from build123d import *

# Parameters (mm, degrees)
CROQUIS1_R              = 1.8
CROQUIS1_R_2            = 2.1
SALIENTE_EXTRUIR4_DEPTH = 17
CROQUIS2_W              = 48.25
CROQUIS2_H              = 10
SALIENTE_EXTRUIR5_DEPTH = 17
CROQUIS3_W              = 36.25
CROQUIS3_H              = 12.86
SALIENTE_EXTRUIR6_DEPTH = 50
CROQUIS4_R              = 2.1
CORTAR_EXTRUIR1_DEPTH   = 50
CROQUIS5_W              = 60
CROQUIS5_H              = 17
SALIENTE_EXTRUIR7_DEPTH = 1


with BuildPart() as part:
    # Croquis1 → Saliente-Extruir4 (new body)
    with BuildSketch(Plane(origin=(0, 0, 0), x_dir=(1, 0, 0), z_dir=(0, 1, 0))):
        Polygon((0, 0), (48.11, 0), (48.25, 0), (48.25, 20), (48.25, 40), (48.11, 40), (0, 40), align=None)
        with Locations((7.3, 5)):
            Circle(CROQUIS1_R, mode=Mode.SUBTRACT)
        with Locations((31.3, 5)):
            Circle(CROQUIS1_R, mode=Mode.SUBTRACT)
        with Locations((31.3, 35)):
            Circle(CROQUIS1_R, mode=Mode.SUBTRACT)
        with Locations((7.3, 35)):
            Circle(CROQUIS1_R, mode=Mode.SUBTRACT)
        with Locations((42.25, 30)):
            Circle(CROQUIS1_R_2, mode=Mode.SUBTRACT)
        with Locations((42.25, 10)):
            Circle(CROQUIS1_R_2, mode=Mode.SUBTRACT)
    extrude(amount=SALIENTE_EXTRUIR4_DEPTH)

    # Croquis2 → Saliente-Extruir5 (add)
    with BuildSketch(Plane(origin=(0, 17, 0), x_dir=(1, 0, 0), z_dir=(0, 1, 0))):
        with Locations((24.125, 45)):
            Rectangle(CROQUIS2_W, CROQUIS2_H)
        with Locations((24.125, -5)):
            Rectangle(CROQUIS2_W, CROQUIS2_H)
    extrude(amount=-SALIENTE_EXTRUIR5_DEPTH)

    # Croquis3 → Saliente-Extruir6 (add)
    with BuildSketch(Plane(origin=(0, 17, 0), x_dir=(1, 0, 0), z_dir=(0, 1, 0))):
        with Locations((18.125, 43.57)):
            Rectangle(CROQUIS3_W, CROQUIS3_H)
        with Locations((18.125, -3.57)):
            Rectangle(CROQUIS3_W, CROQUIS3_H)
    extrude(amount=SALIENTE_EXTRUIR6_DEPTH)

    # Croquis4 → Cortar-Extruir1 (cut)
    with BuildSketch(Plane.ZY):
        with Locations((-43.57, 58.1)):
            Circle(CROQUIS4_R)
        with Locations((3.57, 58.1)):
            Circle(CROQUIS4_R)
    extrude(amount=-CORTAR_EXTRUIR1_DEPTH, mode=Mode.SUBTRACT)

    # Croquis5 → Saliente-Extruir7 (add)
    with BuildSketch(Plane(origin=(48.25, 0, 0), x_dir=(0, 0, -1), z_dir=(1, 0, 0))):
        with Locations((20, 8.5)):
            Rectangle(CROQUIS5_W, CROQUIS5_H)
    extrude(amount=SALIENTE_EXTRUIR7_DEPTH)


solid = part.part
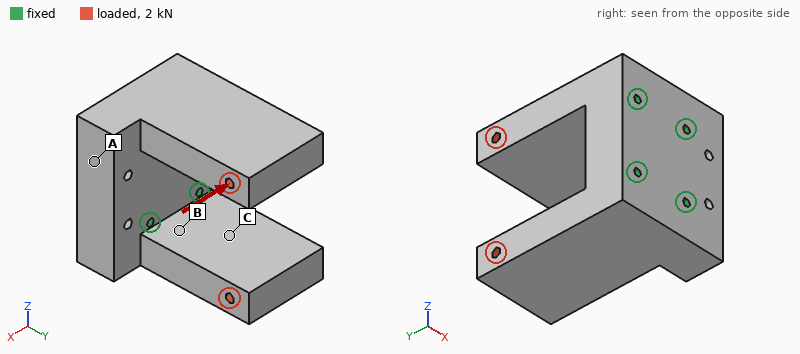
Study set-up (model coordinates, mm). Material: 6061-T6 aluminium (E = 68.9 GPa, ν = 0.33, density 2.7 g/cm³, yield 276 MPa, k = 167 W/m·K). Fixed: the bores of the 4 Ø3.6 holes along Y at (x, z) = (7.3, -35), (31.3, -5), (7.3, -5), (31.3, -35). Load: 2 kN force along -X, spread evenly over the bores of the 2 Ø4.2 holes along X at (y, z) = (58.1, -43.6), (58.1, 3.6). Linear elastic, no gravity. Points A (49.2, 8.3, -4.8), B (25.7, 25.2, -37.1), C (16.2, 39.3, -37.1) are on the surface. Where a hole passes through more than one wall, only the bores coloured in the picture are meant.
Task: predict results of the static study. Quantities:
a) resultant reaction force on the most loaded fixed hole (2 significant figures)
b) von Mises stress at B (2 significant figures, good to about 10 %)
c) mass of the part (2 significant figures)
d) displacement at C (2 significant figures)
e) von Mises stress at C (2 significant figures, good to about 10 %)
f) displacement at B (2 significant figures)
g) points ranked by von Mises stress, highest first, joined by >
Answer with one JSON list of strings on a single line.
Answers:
["1.6 kN", "10 MPa", "260 g", "11 µm", "6.2 MPa", "4.7 µm", "B > C > A"]
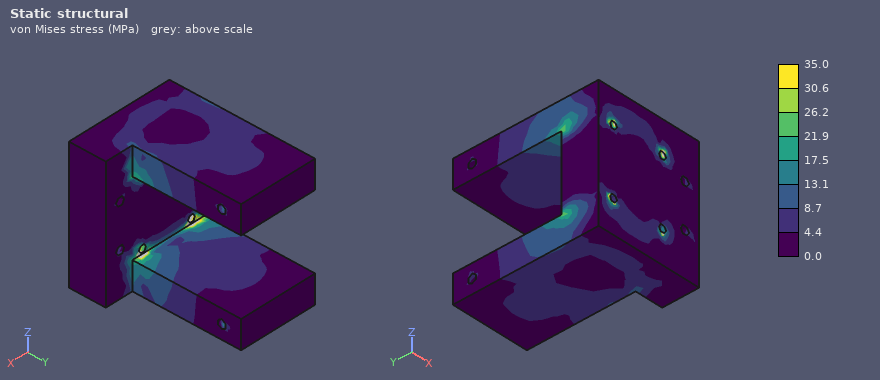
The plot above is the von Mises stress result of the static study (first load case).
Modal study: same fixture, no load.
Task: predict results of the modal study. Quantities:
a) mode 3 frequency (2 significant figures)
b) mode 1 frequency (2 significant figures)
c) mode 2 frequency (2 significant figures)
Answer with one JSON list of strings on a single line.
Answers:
["6300 Hz", "3100 Hz", "3100 Hz"]
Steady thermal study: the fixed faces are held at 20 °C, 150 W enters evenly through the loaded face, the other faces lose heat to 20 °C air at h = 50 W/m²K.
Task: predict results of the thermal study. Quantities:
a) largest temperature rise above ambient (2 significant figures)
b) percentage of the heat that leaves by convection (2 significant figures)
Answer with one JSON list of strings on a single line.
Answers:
["47 K", "12 %"]
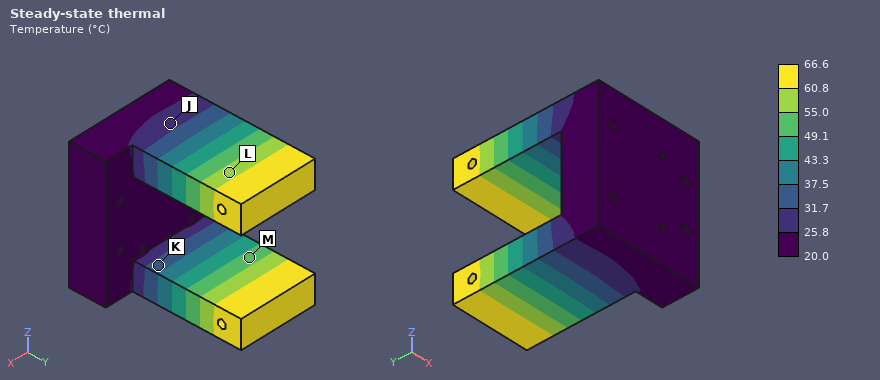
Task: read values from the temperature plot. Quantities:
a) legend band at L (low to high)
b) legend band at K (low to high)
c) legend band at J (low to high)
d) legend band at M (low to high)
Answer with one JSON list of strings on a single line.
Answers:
["55.0 to 60.8 °C", "31.7 to 37.5 °C", "25.8 to 31.7 °C", "49.1 to 55.0 °C"]
